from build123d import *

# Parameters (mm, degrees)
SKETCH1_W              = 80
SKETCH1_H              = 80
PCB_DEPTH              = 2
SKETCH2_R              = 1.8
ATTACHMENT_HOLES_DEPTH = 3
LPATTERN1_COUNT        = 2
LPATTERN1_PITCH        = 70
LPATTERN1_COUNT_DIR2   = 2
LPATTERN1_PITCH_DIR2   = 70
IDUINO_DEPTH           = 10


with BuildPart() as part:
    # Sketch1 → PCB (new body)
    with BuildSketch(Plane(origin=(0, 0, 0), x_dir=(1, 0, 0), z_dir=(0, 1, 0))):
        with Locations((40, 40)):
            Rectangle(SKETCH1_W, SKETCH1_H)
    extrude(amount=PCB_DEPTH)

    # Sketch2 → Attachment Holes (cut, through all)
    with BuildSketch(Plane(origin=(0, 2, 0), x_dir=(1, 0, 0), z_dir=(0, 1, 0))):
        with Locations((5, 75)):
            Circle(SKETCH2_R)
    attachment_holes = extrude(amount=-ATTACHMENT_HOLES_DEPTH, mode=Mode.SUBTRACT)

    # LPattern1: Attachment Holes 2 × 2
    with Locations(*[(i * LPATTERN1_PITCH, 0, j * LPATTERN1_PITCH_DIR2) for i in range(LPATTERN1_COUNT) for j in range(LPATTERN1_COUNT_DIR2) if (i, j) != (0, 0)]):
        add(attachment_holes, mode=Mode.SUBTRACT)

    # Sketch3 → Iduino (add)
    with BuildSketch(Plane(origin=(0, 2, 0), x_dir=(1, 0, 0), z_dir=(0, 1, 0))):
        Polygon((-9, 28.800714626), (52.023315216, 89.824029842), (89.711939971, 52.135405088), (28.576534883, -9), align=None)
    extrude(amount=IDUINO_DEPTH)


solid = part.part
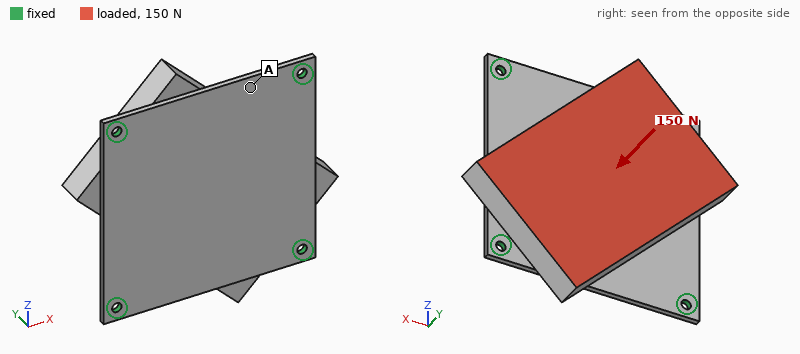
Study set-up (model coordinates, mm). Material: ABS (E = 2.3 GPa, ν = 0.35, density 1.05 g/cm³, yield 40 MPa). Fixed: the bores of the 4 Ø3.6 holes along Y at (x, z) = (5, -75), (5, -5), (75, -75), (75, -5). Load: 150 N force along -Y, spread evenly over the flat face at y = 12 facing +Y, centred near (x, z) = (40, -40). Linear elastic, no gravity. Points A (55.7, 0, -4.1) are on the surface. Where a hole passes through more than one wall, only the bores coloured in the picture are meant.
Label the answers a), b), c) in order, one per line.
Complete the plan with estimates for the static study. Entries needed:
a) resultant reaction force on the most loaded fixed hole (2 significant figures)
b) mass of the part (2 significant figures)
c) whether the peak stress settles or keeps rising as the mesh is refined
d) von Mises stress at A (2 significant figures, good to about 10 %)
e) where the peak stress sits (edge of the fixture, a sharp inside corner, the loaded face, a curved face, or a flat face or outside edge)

a) 99 N
b) 62 g
c) keeps rising
d) 1.5 MPa
e) edge of the fixture
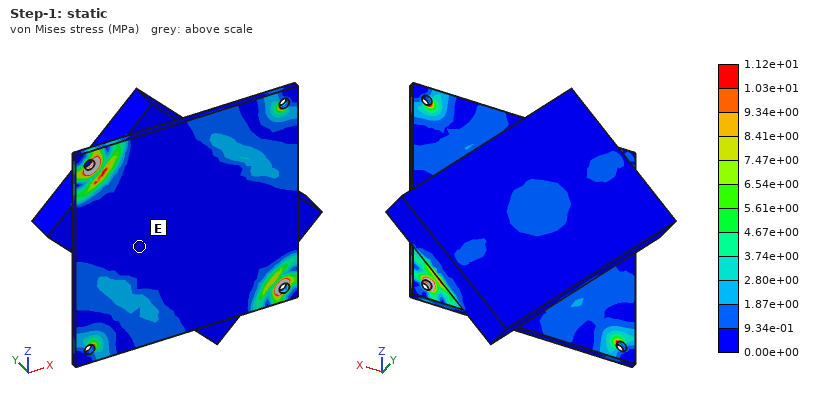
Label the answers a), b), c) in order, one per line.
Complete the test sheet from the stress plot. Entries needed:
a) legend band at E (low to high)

a) 0.00e+00 to 9.34e-01 MPa
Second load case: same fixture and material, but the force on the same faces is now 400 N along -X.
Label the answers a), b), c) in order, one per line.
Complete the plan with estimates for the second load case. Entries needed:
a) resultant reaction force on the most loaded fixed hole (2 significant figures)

a) 130 N
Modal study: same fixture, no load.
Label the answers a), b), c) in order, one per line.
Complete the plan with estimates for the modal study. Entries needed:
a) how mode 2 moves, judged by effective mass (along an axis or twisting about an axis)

a) along Y
